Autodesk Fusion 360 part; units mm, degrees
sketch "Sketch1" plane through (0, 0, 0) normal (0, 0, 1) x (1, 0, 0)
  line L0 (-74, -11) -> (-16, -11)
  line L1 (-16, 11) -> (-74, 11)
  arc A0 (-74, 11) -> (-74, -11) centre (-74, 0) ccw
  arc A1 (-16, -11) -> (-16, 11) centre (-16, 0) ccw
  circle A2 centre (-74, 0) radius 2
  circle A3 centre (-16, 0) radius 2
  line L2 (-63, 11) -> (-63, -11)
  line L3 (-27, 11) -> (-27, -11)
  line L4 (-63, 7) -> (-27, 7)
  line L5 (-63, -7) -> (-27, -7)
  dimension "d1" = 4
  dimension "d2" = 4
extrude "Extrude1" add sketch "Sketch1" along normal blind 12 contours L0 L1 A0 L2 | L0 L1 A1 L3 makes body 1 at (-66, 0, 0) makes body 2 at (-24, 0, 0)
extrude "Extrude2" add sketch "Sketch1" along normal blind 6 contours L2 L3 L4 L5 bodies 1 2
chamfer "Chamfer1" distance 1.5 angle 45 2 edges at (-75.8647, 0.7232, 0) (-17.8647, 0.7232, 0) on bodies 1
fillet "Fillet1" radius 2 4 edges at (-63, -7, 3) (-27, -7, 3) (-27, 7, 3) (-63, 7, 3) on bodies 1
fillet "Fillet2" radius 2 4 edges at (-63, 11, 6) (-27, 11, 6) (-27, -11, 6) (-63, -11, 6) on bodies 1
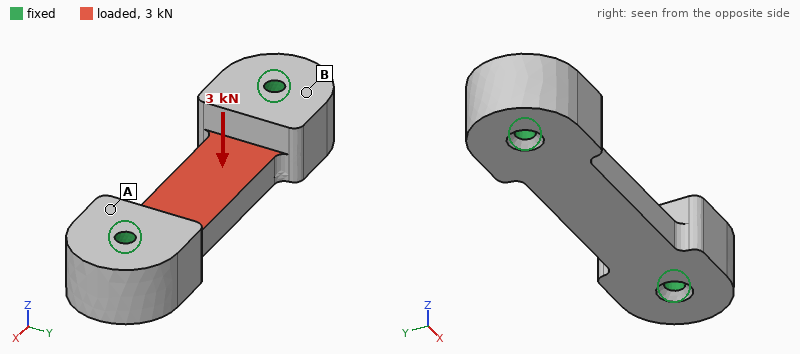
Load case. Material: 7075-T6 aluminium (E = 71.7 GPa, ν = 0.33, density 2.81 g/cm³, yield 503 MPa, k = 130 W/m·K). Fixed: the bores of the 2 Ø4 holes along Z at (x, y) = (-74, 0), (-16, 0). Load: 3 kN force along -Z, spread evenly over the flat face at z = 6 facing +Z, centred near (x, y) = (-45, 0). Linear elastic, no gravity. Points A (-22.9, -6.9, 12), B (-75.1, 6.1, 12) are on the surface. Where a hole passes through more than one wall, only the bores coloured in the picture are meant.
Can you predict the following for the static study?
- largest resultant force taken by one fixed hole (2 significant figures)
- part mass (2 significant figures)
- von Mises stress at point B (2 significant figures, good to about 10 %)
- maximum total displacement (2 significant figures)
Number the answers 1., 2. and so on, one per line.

1. 1.7 kN
2. 37 g
3. 19 MPa
4. 57 µm
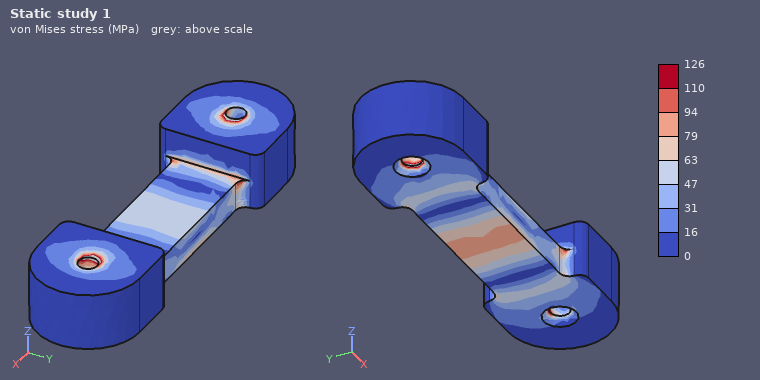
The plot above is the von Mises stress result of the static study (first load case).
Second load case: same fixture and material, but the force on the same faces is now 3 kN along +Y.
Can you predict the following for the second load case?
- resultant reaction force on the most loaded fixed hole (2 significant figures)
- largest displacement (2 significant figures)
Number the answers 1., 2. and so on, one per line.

1. 1.5 kN
2. 47 µm
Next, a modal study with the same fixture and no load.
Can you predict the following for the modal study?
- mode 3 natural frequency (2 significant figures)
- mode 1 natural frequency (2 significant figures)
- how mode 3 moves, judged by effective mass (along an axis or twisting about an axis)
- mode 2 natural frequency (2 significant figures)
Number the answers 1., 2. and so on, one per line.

1. 26 kHz
2. 14 kHz
3. twisting about X
4. 14 kHz
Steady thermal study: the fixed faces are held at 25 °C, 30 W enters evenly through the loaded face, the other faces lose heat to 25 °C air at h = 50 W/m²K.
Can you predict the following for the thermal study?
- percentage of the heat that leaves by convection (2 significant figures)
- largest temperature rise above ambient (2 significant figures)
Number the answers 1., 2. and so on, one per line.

1. 3.6 %
2. 20 K
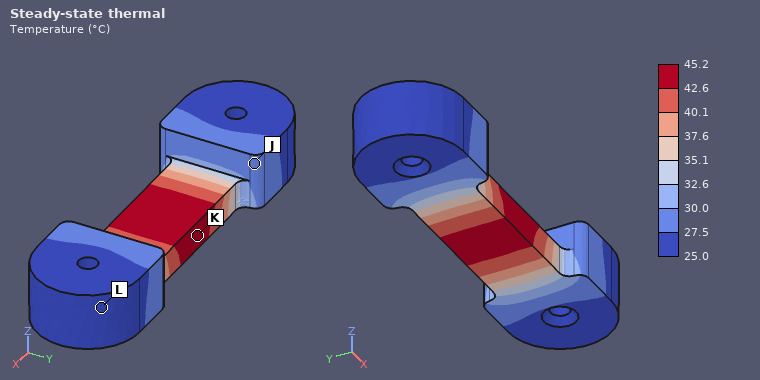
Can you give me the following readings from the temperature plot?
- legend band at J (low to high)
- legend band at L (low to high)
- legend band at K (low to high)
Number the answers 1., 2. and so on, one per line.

1. 27.5 to 30.0 °C
2. 25.0 to 27.5 °C
3. 42.6 to 45.2 °C
